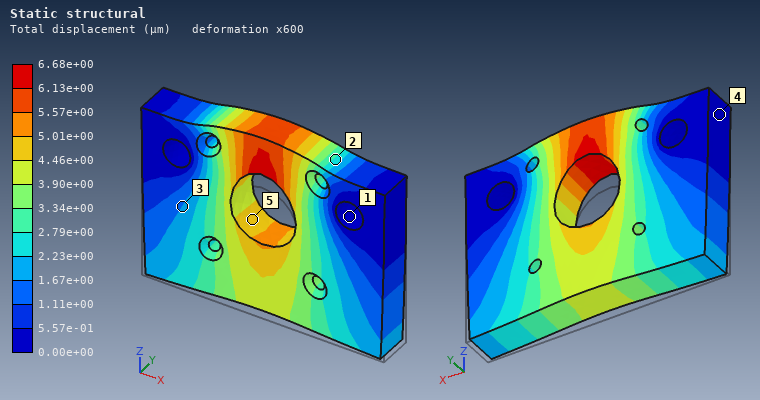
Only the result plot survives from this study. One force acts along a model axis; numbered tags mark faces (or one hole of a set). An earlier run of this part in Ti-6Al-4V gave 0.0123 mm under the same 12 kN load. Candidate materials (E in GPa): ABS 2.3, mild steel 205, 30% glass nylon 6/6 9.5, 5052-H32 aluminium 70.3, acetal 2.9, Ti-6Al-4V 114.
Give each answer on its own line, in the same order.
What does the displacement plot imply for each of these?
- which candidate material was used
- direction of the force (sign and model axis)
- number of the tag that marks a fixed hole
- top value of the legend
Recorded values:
mild steel
+Z
1
6.68e+00 µm
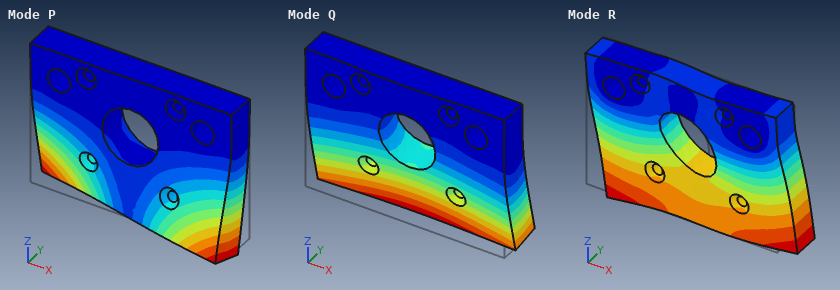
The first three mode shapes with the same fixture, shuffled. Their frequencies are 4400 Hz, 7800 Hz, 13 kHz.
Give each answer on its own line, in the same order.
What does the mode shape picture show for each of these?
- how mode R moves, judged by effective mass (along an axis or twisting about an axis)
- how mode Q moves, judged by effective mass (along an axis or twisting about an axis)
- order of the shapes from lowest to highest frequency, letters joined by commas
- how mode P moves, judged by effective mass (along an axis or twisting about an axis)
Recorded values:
along X
along Y
Q, P, R
twisting about Z
